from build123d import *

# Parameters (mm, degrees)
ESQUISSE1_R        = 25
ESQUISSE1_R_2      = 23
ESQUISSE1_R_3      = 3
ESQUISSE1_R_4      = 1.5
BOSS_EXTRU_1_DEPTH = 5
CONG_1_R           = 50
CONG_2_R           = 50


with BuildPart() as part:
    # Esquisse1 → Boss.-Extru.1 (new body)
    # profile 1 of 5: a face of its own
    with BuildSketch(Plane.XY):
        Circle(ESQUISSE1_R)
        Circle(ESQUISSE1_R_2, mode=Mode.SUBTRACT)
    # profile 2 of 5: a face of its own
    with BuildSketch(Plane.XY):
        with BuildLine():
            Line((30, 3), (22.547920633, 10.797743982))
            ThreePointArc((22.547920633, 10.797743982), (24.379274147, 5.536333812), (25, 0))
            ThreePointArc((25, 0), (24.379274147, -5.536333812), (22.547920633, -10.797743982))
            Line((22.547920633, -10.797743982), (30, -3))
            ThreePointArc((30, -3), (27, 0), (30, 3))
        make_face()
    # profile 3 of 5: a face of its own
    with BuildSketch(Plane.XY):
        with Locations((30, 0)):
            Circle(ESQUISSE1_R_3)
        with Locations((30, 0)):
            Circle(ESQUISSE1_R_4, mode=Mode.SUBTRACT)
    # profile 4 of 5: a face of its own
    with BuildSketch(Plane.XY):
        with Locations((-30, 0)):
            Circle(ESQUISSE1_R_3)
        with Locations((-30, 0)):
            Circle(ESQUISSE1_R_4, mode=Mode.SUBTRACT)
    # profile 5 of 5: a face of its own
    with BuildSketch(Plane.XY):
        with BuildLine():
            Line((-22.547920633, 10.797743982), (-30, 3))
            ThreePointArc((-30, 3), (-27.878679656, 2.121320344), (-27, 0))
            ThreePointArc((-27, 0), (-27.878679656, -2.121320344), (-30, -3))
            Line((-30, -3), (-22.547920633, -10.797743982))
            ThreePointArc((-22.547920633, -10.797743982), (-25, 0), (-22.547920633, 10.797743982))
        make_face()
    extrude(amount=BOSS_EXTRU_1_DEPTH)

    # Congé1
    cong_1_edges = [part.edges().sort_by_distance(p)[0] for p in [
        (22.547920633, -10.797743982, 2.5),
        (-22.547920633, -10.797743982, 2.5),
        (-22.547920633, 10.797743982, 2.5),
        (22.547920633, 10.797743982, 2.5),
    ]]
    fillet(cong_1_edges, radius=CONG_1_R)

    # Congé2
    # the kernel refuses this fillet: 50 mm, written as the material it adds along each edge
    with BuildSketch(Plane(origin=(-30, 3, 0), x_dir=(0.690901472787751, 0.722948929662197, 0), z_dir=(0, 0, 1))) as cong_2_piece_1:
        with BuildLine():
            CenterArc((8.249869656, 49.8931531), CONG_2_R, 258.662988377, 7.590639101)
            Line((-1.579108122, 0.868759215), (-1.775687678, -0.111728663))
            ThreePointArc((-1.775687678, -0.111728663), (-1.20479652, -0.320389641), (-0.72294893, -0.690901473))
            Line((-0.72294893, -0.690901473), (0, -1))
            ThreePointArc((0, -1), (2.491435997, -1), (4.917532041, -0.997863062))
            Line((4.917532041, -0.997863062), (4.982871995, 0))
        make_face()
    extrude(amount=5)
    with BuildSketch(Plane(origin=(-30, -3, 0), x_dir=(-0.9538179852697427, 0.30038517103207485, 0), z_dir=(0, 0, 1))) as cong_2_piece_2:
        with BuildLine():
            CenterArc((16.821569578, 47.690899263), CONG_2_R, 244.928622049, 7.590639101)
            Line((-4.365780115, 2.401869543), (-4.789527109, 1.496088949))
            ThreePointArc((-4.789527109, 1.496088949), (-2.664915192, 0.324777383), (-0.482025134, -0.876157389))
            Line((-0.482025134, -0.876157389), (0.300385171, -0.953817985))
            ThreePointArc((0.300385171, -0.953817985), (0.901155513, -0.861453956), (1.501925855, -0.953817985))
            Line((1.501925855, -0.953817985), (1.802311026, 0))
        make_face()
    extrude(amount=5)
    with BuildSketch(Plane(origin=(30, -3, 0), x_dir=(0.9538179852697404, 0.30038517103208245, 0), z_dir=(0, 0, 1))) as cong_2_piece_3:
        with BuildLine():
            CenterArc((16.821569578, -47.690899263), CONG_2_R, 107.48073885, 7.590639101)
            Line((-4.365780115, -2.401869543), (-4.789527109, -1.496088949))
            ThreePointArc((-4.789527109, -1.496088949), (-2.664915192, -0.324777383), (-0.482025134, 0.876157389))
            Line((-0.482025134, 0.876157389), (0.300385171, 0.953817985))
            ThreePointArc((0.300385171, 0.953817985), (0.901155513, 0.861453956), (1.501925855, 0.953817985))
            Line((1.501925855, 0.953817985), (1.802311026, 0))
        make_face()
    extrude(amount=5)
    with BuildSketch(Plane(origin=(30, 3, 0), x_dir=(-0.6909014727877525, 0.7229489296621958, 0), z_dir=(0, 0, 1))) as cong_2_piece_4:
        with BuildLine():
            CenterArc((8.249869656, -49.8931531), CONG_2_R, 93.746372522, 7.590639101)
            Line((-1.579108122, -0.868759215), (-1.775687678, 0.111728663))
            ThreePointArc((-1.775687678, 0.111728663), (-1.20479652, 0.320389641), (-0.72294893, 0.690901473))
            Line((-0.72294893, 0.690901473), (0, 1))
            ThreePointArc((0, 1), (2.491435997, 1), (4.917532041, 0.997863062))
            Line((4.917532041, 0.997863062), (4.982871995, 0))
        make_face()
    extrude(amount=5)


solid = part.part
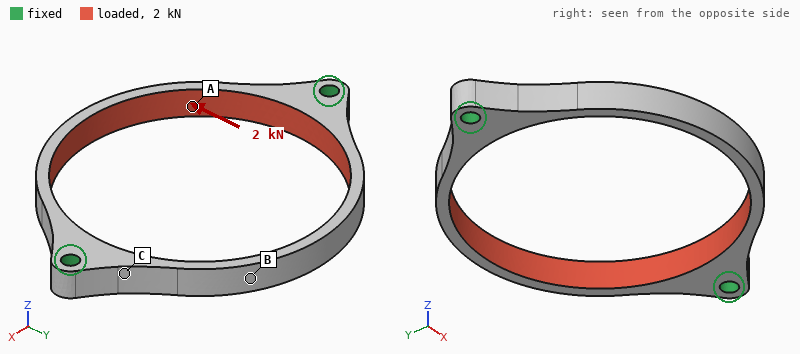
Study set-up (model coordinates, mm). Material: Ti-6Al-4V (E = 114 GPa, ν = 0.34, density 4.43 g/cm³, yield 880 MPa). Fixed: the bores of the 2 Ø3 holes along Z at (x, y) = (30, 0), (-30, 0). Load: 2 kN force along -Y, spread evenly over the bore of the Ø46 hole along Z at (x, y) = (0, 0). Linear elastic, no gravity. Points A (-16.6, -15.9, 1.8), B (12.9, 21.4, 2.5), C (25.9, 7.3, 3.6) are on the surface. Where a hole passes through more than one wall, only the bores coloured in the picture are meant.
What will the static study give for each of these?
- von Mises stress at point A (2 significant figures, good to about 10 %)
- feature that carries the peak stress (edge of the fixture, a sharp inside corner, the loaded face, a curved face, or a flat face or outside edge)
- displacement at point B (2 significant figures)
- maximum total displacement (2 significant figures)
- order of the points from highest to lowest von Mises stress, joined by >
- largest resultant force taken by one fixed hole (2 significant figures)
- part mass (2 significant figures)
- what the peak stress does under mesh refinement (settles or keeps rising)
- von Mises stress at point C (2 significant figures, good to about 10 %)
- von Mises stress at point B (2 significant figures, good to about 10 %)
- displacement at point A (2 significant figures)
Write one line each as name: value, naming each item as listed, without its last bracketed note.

von Mises stress at point A: 69 MPa
feature that carries the peak stress: edge of the fixture
displacement at point B: 9.5 µm
maximum total displacement: 26 µm
order of the points from highest to lowest von Mises stress, joined by >: A > C > B
largest resultant force taken by one fixed hole: 1.0 kN
part mass: 10 g
what the peak stress does under mesh refinement: keeps rising
von Mises stress at point C: 43 MPa
von Mises stress at point B: 15 MPa
displacement at point A: 6.1 µm
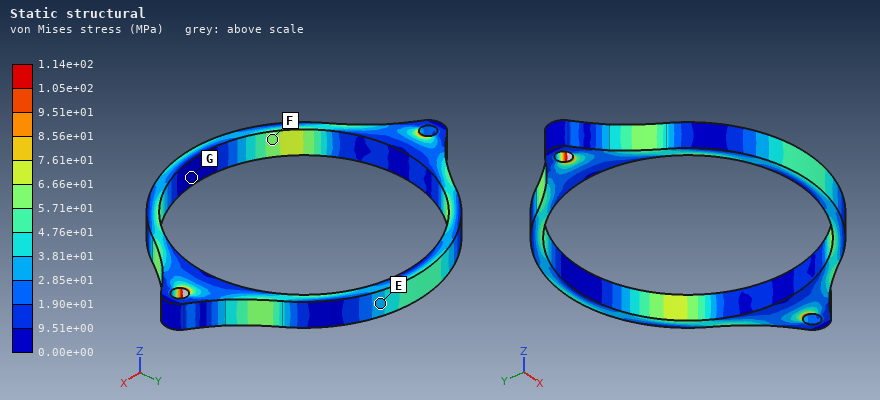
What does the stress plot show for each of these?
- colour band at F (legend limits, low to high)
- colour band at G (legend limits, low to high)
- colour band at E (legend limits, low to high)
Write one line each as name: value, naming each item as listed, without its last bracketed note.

colour band at F: 5.71e+01 to 6.66e+01 MPa
colour band at G: 0.00e+00 to 9.51e+00 MPa
colour band at E: 2.85e+01 to 3.81e+01 MPa
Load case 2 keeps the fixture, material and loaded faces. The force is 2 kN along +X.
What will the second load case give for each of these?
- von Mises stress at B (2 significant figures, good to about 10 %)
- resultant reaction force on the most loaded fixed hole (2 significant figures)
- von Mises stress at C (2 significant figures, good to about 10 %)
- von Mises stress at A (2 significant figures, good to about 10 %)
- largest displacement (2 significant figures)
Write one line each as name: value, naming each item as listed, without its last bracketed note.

von Mises stress at B: 200 MPa
resultant reaction force on the most loaded fixed hole: 1.0 kN
von Mises stress at C: 200 MPa
von Mises stress at A: 150 MPa
largest displacement: 0.19 mm
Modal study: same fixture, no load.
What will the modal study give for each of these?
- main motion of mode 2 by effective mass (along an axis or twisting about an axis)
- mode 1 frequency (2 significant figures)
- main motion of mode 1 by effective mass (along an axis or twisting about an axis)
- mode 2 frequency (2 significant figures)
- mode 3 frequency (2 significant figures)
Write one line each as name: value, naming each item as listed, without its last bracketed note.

main motion of mode 2 by effective mass: along Z
mode 1 frequency: 4200 Hz
main motion of mode 1 by effective mass: twisting about X
mode 2 frequency: 4400 Hz
mode 3 frequency: 6000 Hz
